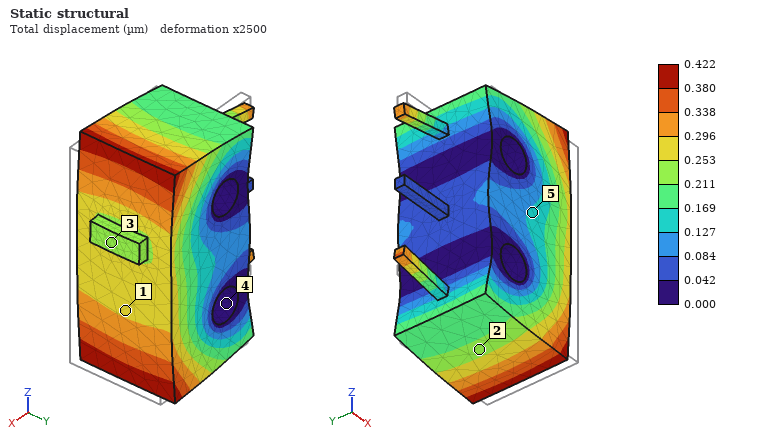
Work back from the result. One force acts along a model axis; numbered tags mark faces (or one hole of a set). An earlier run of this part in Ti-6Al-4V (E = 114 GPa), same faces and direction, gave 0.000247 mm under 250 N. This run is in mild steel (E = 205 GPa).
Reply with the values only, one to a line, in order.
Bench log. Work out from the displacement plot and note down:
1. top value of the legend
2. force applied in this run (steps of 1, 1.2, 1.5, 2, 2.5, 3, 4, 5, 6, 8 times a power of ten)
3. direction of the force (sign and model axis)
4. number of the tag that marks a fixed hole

0.422 µm
800 N
-X
4
